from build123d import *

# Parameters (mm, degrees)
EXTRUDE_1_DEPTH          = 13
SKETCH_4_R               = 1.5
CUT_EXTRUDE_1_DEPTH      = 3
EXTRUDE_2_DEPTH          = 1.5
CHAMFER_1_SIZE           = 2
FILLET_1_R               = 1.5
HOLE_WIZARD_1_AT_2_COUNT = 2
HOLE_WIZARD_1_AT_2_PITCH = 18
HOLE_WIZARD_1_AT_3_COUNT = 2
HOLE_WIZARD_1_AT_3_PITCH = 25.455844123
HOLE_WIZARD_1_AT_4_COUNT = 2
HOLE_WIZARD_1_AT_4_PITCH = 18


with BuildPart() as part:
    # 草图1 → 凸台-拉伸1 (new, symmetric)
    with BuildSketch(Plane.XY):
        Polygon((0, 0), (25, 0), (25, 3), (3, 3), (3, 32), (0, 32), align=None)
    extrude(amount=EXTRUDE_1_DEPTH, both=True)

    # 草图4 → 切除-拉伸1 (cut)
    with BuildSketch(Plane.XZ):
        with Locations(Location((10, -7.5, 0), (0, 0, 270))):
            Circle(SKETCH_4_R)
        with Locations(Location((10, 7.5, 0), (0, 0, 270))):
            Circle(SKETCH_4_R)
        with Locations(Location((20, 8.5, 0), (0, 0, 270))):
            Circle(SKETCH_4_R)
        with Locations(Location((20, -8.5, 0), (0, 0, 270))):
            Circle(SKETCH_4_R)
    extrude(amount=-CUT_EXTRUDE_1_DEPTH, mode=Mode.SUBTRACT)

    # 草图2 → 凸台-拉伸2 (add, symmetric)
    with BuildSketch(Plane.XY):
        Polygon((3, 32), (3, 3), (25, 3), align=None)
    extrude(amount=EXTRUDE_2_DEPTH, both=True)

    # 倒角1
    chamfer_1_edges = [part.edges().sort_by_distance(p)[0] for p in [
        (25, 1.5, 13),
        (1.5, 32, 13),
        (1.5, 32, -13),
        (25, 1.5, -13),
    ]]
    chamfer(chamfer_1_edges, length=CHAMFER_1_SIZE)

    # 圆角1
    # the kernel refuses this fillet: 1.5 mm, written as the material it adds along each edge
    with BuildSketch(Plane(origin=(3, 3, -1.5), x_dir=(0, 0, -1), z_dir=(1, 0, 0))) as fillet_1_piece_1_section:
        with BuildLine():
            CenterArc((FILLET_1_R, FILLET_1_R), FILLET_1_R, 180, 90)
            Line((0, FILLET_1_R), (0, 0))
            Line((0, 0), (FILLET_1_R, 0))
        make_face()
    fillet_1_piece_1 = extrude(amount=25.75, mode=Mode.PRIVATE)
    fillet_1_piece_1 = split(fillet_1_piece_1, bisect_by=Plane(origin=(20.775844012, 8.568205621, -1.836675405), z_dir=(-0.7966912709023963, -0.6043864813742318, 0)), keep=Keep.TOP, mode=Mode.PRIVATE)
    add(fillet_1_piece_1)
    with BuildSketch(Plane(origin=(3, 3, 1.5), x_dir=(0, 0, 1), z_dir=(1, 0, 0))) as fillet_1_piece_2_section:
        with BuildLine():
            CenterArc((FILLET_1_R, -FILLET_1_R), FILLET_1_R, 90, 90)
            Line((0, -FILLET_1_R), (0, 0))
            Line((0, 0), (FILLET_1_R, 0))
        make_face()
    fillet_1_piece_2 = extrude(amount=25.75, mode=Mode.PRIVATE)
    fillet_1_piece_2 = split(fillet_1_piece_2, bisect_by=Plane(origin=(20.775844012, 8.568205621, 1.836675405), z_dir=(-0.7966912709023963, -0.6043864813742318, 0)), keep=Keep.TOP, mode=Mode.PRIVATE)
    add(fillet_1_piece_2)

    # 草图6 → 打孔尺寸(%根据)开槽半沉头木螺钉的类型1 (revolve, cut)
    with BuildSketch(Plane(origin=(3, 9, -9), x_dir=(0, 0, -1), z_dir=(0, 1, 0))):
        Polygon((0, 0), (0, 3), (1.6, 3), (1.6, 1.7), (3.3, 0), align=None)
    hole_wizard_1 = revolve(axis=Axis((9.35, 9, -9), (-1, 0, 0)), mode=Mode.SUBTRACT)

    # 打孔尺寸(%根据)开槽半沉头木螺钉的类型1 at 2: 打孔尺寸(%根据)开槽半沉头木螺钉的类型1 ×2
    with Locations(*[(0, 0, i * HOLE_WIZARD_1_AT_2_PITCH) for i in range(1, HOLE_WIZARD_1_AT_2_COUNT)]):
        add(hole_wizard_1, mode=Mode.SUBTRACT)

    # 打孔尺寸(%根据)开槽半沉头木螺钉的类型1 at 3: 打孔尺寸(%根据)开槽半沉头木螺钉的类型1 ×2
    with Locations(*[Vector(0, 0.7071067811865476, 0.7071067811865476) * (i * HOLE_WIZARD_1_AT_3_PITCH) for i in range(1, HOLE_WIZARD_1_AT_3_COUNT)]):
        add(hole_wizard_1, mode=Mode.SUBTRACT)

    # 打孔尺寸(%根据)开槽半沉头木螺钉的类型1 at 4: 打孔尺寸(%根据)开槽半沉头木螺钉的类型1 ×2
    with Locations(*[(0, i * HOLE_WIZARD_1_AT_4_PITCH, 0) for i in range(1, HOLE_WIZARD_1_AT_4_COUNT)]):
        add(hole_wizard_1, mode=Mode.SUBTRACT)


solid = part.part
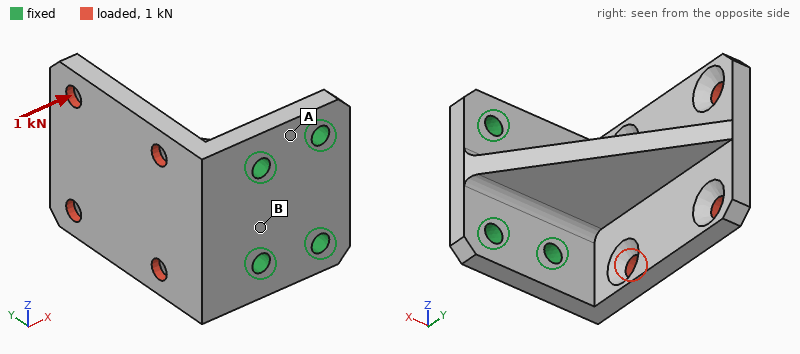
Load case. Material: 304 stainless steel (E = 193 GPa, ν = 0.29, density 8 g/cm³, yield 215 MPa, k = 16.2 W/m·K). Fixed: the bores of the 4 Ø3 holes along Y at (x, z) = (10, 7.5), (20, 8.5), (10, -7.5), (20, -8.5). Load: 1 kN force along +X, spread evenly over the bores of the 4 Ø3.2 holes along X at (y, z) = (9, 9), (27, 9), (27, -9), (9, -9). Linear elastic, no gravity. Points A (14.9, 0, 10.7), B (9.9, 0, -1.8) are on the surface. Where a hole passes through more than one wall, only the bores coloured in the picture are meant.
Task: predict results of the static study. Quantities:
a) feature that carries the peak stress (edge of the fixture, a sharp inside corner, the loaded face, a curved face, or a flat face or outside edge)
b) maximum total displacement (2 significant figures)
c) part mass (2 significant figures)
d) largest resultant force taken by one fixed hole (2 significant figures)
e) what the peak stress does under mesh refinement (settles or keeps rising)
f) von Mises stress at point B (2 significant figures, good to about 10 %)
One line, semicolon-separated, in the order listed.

edge of the fixture; 53 µm; 39 g; 630 N; keeps rising; 39 MPa
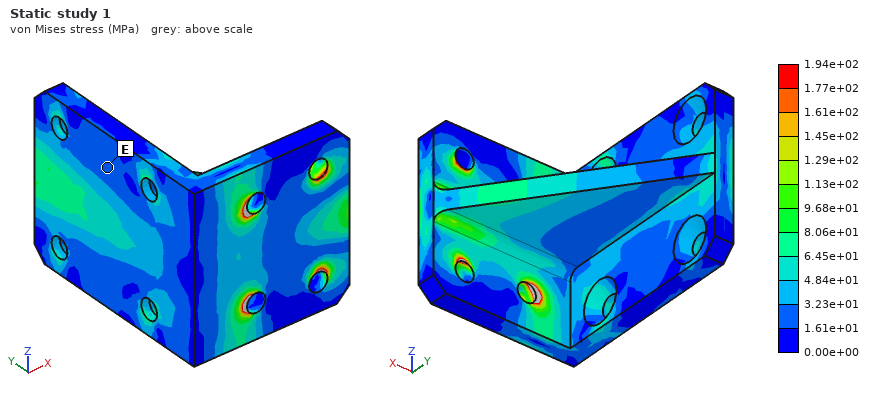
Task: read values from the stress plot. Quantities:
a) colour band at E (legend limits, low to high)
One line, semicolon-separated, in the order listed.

1.61e+01 to 3.23e+01 MPa
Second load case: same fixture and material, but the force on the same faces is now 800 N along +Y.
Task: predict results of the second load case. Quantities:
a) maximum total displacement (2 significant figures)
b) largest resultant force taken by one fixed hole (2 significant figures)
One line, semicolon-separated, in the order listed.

21 µm; 600 N
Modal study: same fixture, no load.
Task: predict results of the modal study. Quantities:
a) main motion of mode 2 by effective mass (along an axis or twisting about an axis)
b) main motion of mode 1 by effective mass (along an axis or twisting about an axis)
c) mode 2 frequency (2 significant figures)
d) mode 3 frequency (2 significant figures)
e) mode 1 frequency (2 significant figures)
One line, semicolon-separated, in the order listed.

along X; along Z; 6200 Hz; 8200 Hz; 5500 Hz
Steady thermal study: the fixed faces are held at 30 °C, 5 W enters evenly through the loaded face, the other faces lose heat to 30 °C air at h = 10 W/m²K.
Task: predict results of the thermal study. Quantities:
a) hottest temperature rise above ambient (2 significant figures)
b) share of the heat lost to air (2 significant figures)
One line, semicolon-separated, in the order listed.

67 K; 20 %
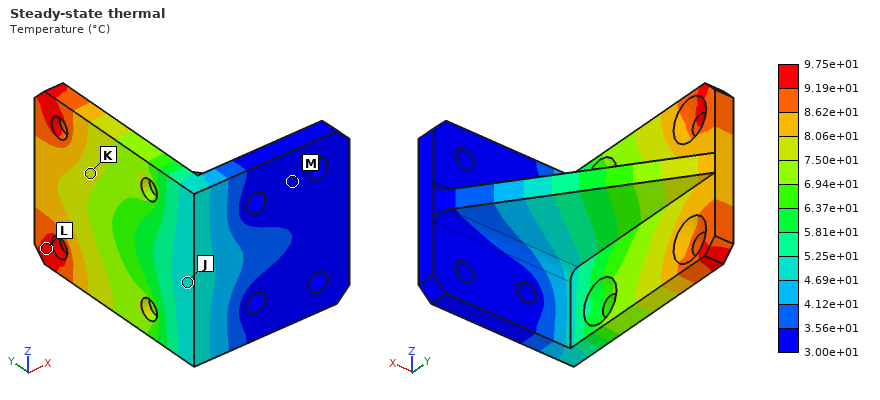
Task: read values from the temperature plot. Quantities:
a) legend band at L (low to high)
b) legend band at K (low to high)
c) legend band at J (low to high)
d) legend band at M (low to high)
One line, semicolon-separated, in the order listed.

9.19e+01 to 9.75e+01 °C; 7.50e+01 to 8.06e+01 °C; 4.69e+01 to 5.25e+01 °C; 3.00e+01 to 3.56e+01 °C
